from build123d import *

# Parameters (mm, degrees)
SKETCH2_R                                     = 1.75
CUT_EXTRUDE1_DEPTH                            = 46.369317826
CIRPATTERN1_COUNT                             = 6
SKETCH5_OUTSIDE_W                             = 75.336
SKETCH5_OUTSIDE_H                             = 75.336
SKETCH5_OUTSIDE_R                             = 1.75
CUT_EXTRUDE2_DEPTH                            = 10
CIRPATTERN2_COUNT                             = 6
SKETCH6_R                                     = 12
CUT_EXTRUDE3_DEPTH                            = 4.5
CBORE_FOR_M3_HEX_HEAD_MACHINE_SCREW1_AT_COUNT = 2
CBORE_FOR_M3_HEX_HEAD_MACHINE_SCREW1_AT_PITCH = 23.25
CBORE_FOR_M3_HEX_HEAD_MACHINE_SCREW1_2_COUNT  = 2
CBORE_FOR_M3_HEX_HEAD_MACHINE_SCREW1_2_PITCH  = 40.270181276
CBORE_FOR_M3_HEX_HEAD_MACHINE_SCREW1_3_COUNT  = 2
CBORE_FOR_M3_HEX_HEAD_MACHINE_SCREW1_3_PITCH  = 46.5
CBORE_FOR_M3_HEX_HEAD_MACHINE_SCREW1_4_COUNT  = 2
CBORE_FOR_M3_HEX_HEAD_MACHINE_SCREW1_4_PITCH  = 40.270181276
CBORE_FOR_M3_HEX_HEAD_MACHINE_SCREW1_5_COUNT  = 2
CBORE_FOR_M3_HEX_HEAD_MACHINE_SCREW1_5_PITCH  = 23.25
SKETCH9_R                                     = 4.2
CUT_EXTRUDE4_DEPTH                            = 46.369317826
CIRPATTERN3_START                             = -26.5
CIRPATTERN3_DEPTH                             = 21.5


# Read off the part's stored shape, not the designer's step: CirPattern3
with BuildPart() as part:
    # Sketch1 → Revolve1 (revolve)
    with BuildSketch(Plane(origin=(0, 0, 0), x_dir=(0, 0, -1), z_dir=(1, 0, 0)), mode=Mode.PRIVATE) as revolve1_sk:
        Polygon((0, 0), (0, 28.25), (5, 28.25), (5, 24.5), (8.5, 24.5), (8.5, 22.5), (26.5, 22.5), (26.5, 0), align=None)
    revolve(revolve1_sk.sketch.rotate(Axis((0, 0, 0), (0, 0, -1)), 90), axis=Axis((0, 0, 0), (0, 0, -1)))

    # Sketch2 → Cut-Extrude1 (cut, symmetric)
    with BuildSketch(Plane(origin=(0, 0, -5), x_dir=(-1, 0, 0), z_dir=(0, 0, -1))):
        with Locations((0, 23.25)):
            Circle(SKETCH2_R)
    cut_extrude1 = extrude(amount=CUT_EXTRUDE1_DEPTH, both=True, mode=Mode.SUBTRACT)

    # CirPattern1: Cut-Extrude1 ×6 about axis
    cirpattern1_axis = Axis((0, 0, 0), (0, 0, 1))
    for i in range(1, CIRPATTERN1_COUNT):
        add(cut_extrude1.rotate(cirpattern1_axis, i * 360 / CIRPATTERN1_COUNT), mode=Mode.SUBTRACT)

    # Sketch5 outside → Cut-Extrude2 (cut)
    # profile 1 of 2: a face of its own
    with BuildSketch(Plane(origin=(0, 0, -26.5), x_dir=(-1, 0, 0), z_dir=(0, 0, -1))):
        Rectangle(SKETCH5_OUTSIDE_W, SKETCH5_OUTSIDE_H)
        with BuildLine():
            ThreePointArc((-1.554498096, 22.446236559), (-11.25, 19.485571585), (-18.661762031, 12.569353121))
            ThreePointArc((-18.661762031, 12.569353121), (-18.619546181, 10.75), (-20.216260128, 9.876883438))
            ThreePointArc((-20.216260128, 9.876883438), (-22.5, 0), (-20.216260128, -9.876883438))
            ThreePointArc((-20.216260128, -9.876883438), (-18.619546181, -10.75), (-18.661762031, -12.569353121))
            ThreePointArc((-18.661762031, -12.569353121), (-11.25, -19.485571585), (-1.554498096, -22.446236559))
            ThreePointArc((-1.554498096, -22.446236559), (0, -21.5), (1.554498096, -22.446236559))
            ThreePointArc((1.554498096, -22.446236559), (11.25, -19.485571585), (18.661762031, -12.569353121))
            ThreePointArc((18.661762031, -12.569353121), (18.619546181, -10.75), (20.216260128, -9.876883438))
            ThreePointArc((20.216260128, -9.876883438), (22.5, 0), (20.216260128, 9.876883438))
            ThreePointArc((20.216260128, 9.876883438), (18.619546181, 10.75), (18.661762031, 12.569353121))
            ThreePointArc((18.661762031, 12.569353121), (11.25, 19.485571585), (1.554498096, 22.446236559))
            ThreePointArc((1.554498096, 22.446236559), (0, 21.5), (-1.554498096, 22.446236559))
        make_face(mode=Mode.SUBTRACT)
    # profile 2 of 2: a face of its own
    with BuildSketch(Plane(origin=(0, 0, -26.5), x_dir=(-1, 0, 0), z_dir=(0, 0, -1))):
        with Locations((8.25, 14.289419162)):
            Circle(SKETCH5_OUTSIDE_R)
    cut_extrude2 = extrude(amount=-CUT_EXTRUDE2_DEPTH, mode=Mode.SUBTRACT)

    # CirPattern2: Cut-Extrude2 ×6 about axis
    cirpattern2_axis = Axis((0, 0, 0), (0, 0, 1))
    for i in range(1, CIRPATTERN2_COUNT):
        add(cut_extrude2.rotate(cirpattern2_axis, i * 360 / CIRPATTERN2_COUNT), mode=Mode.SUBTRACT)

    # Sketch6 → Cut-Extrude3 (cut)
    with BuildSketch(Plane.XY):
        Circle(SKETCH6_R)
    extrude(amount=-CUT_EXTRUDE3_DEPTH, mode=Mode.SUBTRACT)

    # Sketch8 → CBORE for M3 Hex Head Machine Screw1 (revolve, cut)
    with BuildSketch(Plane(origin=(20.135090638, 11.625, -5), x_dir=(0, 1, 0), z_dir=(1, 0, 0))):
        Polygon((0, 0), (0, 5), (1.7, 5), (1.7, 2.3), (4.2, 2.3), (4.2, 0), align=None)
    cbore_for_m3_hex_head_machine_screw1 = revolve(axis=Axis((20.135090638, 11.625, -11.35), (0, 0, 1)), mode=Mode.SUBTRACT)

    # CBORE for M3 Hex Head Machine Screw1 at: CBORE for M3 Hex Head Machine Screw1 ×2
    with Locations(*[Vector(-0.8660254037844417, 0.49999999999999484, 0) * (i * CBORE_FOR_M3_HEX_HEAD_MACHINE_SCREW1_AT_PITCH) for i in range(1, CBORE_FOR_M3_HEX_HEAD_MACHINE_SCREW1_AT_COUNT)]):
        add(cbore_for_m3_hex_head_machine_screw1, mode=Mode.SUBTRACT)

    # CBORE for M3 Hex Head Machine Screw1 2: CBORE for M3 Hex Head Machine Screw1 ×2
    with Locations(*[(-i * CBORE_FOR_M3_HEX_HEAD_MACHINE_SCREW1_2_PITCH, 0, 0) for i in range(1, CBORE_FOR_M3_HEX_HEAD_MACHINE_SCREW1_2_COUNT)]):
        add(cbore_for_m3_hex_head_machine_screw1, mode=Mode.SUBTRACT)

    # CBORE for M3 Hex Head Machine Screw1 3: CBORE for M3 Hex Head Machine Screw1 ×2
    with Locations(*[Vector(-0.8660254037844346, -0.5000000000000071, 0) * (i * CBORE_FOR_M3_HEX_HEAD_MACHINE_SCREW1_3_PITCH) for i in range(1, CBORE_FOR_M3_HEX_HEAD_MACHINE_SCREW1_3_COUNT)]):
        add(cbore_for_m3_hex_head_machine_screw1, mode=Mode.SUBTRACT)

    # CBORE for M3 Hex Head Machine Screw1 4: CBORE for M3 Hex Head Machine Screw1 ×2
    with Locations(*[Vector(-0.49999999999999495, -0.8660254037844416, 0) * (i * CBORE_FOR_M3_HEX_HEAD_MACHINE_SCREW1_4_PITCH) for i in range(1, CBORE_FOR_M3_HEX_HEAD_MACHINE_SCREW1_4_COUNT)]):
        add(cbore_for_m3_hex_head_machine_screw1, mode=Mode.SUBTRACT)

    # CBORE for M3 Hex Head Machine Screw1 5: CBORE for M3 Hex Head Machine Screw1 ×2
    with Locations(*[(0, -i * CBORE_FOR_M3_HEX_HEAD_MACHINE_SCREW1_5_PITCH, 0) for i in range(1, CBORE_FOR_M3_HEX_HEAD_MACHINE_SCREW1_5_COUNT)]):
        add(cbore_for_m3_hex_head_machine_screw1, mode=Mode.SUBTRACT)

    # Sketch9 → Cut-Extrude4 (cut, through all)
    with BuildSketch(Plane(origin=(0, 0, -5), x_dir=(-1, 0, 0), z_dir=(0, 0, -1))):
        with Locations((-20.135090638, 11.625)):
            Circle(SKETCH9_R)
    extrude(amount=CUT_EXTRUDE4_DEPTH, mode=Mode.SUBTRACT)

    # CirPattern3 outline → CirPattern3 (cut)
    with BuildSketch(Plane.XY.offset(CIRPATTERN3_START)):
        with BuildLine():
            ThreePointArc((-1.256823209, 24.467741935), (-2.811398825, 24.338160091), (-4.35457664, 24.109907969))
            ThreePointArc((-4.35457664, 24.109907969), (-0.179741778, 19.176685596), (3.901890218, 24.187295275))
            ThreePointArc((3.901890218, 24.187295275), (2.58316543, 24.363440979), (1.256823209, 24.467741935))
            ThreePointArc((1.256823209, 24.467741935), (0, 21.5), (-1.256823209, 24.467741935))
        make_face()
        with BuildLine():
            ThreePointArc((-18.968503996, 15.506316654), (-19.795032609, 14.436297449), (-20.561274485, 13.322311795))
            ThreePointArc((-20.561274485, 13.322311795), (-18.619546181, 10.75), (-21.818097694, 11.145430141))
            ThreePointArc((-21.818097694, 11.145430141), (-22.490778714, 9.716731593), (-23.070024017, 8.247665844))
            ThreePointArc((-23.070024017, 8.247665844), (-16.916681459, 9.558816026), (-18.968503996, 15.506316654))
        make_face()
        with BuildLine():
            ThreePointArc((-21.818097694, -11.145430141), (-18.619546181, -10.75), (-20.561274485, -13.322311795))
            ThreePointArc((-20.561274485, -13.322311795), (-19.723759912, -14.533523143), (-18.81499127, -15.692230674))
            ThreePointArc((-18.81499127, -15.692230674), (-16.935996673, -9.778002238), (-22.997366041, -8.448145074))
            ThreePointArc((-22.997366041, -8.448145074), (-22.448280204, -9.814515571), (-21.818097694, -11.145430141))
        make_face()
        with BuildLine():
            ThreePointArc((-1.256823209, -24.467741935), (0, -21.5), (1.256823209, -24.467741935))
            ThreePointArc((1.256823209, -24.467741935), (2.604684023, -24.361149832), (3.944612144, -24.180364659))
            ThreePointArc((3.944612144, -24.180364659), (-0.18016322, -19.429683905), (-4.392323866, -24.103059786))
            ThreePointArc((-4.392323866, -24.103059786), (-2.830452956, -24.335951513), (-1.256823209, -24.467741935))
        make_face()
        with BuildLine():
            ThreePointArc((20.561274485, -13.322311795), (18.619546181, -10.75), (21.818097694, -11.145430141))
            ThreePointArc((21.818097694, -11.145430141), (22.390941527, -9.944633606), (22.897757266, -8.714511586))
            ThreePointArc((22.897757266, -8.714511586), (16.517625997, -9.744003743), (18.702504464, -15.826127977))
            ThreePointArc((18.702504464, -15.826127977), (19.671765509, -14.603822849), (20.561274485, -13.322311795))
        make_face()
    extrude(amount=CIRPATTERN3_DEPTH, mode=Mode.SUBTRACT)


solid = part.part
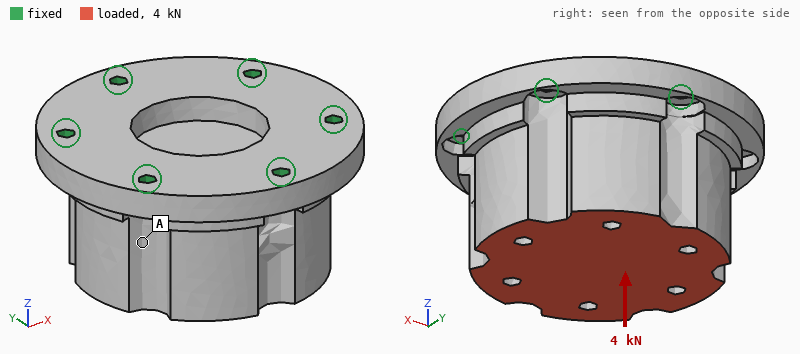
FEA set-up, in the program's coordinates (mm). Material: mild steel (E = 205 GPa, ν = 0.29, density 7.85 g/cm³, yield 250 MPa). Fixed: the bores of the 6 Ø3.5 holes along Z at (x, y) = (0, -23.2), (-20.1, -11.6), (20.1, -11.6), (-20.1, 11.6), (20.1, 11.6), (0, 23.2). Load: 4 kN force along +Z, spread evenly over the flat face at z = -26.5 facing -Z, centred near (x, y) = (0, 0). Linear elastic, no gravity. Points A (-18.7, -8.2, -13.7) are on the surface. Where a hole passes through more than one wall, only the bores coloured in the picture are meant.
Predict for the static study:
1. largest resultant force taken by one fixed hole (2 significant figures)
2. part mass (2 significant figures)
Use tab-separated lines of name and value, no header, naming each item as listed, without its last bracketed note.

largest resultant force taken by one fixed hole	740 N
part mass	330 g
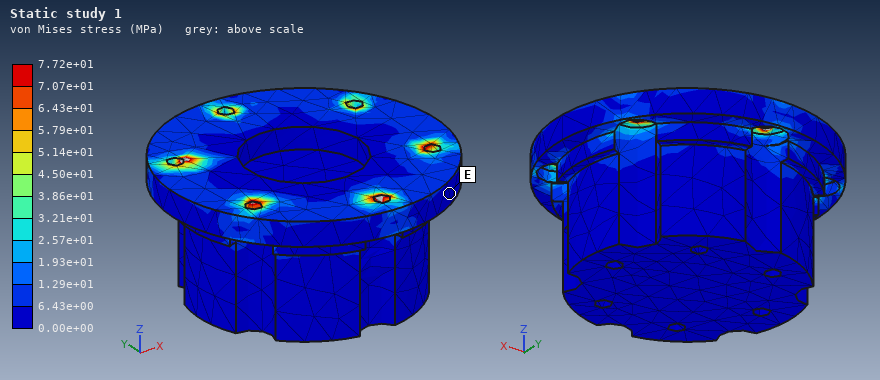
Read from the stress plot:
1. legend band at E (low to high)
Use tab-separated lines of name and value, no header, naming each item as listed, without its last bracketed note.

legend band at E	0.00e+00 to 6.43e+00 MPa
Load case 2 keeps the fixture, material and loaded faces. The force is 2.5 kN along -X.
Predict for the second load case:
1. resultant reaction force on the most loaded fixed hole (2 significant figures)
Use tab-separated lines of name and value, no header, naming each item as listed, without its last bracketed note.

resultant reaction force on the most loaded fixed hole	960 N
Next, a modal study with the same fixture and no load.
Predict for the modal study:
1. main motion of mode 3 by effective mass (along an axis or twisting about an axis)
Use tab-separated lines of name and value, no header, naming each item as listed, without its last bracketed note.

main motion of mode 3 by effective mass	along Z
